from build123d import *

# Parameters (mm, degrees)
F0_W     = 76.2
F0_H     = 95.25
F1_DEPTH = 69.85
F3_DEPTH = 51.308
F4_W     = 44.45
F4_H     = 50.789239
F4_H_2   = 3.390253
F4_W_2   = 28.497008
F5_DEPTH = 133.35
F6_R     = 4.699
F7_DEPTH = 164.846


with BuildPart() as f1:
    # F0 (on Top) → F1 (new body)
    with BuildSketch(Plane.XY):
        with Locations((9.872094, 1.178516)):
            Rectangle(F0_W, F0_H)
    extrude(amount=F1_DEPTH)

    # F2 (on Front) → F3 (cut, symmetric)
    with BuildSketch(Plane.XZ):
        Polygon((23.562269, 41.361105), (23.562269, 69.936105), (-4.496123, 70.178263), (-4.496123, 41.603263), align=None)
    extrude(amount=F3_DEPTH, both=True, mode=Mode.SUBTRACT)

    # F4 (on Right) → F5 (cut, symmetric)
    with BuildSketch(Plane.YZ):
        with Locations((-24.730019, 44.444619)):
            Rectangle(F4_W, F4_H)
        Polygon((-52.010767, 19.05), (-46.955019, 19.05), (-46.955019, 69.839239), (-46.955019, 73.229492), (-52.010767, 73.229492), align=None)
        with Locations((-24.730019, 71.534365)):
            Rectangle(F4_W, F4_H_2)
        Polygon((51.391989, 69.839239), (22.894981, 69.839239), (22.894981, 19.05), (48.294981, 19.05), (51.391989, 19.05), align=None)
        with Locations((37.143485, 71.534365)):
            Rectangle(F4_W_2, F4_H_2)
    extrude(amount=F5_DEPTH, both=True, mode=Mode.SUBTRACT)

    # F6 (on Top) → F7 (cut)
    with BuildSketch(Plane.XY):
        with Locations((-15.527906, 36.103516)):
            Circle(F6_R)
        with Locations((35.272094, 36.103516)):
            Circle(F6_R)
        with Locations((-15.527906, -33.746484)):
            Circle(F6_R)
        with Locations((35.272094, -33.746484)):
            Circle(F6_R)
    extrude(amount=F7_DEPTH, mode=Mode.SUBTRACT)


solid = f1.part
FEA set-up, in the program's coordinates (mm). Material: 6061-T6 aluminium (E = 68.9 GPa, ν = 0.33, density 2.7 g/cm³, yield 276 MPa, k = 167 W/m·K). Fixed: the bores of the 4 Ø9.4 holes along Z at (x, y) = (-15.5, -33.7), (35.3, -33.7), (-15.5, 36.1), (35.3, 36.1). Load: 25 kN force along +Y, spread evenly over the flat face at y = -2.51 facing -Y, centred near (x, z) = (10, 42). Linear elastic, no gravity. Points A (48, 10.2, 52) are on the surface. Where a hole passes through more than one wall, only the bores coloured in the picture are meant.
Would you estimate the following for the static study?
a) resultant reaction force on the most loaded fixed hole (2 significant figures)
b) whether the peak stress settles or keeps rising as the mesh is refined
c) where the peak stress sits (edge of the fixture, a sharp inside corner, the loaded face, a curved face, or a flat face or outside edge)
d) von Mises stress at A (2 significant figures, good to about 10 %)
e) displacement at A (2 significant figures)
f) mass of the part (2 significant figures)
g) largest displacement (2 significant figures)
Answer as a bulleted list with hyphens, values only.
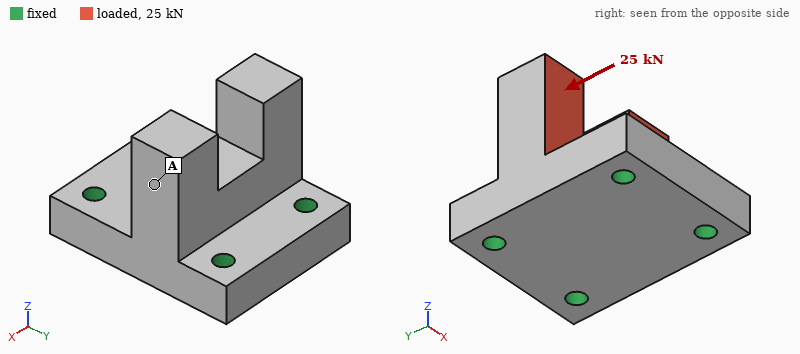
- 10 kN
- keeps rising
- edge of the fixture
- 16 MPa
- 0.093 mm
- 570 g
- 0.15 mm
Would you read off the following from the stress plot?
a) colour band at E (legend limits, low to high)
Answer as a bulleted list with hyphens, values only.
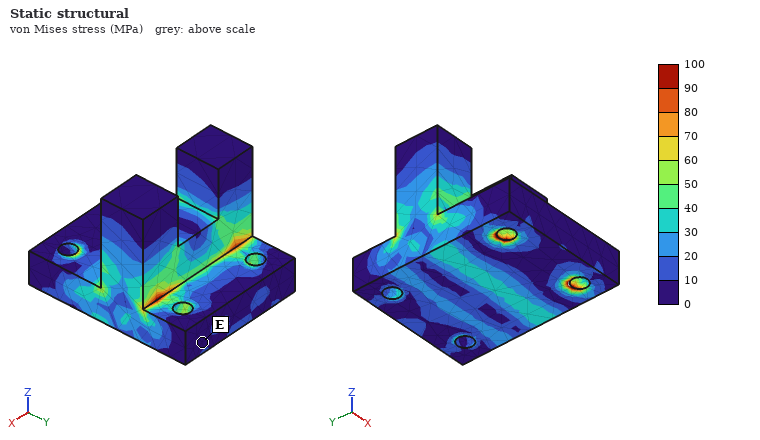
- 0 to 10 MPa
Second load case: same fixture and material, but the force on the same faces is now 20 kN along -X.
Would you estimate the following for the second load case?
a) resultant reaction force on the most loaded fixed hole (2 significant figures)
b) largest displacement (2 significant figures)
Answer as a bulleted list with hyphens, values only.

- 11 kN
- 0.11 mm
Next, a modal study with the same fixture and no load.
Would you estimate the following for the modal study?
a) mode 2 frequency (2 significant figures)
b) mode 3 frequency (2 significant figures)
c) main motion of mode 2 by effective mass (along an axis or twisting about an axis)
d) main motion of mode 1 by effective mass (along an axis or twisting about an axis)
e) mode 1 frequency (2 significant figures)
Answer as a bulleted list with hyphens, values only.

- 6000 Hz
- 6800 Hz
- along X
- along Y
- 5500 Hz
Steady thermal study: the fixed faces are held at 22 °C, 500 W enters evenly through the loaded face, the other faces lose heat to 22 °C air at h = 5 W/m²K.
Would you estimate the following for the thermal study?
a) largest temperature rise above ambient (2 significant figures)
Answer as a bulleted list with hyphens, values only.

- 85 K
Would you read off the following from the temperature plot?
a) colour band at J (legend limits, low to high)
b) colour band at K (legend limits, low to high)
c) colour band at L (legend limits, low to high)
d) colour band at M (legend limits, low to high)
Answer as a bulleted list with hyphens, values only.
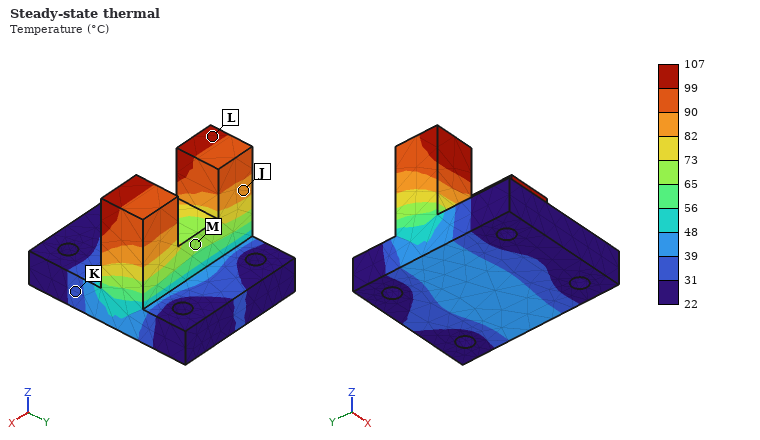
- 82 to 90 °C
- 31 to 39 °C
- 99 to 107 °C
- 65 to 73 °C
